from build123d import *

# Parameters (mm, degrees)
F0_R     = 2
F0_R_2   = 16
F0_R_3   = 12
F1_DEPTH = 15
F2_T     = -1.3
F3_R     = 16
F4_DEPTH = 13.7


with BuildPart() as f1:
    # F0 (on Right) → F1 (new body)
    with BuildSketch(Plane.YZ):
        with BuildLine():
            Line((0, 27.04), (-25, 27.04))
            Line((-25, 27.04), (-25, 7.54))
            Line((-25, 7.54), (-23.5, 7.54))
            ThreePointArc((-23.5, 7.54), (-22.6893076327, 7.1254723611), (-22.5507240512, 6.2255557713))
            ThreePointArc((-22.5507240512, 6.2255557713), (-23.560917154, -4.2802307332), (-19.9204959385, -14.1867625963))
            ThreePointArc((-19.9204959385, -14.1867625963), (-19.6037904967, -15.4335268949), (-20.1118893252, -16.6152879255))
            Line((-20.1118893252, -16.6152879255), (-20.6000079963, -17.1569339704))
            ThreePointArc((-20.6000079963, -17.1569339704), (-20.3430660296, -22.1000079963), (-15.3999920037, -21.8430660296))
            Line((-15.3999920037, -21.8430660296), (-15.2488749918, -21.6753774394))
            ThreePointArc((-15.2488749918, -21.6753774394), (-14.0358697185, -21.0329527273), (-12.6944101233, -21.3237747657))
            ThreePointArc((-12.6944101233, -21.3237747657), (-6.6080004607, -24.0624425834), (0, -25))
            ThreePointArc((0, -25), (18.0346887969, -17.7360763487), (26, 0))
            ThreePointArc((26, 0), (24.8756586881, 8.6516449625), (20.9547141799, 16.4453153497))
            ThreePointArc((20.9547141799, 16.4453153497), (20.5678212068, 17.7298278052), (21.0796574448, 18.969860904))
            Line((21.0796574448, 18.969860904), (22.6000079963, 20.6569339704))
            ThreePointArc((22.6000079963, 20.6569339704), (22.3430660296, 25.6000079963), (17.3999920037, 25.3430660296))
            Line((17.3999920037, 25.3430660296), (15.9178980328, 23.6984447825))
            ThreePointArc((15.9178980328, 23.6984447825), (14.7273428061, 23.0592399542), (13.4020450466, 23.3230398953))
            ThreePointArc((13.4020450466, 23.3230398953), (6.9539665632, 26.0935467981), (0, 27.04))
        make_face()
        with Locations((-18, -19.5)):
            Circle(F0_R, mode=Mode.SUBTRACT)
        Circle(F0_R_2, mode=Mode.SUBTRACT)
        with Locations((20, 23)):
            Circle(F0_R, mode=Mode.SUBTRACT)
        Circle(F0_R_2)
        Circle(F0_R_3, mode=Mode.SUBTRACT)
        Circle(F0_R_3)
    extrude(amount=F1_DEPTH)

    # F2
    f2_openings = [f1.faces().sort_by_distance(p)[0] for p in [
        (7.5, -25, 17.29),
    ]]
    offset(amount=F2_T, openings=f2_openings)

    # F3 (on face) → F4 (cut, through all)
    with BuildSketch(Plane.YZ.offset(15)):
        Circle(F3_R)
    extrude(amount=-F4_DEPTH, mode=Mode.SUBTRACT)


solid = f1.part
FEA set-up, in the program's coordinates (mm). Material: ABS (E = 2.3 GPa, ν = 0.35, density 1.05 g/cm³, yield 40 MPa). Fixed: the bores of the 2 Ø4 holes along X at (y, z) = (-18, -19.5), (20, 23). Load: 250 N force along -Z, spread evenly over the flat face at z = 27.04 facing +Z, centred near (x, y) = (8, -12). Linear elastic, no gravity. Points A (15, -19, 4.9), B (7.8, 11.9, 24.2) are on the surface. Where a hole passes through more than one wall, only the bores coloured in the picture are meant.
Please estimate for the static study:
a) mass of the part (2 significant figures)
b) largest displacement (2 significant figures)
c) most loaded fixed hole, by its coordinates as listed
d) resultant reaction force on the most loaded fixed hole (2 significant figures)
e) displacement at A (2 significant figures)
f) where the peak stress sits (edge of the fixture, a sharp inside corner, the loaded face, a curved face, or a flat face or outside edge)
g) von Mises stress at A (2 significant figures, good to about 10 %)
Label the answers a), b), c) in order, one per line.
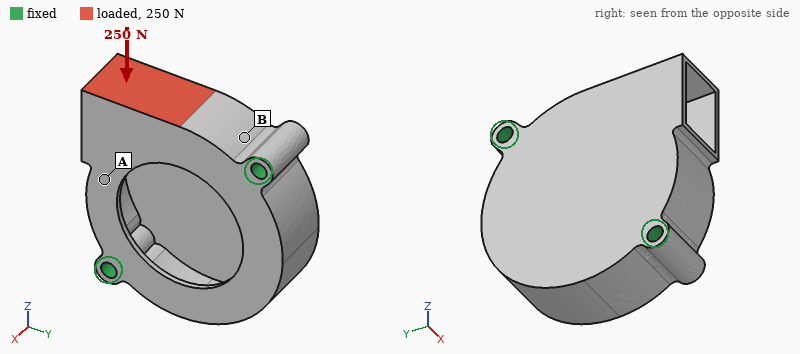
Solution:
a) 8.2 g
b) 0.52 mm
c) (-18, -19.5)
d) 180 N
e) 0.13 mm
f) the loaded face
g) 11 MPa
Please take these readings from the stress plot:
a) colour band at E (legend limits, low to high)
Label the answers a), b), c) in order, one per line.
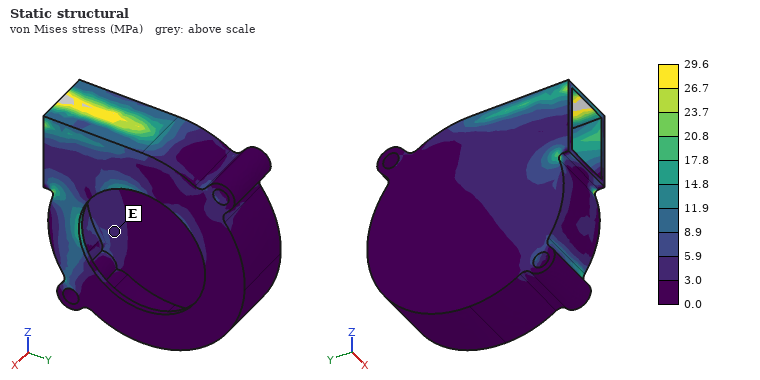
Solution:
a) 3.0 to 5.9 MPa
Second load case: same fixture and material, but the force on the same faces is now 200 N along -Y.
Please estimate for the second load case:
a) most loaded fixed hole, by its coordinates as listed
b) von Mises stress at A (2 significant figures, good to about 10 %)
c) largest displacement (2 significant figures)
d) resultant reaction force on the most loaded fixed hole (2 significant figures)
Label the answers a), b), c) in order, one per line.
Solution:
a) (20, 23)
b) 1.4 MPa
c) 0.14 mm
d) 190 N
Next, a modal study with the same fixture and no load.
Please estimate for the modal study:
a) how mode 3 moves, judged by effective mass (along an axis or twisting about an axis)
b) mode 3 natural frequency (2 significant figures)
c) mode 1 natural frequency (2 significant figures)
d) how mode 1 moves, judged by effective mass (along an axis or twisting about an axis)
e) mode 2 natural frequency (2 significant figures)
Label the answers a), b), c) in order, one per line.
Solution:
a) along X
b) 2400 Hz
c) 1300 Hz
d) along X
e) 1800 Hz
